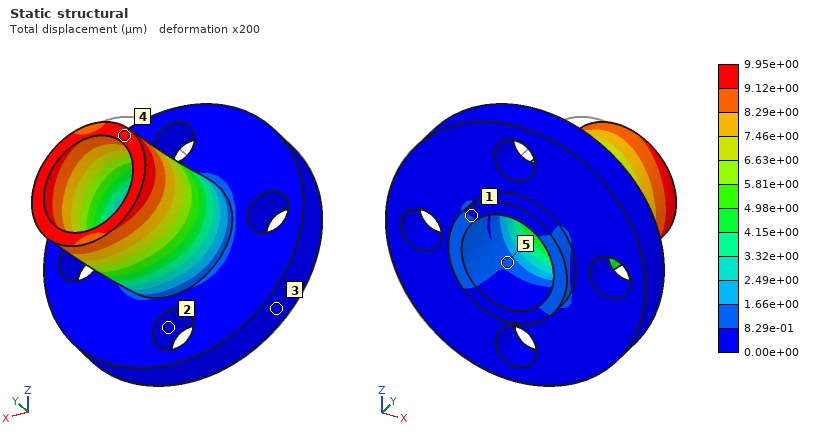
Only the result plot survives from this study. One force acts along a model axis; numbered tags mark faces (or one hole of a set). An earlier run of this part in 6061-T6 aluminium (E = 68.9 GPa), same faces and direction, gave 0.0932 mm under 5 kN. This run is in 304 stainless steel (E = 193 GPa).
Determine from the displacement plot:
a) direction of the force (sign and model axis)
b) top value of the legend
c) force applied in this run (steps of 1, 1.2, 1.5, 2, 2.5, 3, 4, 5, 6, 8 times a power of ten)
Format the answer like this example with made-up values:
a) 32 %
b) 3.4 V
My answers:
a) +X
b) 9.95e+00 µm
c) 1.5 kN
